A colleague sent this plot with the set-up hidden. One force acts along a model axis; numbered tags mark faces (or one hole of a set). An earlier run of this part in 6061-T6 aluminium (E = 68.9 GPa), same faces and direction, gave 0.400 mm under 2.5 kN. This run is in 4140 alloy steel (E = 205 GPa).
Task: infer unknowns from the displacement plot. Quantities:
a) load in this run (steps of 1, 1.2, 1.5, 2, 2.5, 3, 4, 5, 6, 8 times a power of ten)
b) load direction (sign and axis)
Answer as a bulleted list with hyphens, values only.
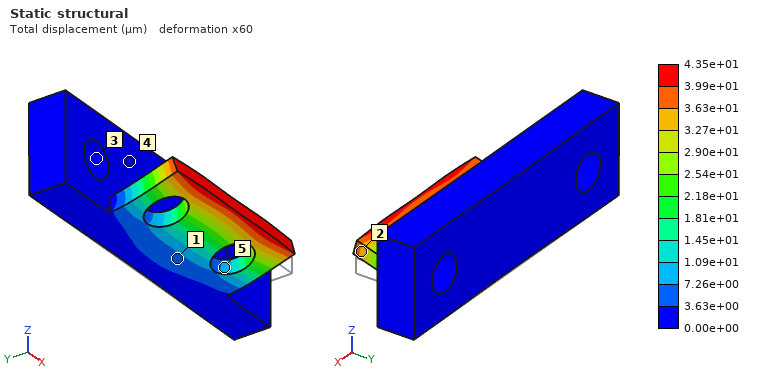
- 800 N
- +Z
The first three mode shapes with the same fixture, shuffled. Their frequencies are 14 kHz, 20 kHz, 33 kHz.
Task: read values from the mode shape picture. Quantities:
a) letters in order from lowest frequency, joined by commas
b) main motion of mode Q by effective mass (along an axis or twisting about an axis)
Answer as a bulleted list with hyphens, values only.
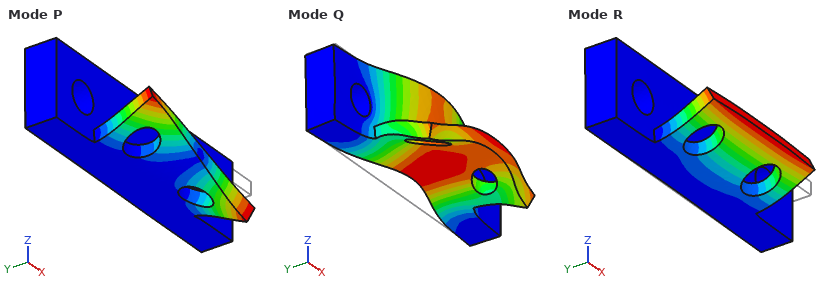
- R, P, Q
- along Y
